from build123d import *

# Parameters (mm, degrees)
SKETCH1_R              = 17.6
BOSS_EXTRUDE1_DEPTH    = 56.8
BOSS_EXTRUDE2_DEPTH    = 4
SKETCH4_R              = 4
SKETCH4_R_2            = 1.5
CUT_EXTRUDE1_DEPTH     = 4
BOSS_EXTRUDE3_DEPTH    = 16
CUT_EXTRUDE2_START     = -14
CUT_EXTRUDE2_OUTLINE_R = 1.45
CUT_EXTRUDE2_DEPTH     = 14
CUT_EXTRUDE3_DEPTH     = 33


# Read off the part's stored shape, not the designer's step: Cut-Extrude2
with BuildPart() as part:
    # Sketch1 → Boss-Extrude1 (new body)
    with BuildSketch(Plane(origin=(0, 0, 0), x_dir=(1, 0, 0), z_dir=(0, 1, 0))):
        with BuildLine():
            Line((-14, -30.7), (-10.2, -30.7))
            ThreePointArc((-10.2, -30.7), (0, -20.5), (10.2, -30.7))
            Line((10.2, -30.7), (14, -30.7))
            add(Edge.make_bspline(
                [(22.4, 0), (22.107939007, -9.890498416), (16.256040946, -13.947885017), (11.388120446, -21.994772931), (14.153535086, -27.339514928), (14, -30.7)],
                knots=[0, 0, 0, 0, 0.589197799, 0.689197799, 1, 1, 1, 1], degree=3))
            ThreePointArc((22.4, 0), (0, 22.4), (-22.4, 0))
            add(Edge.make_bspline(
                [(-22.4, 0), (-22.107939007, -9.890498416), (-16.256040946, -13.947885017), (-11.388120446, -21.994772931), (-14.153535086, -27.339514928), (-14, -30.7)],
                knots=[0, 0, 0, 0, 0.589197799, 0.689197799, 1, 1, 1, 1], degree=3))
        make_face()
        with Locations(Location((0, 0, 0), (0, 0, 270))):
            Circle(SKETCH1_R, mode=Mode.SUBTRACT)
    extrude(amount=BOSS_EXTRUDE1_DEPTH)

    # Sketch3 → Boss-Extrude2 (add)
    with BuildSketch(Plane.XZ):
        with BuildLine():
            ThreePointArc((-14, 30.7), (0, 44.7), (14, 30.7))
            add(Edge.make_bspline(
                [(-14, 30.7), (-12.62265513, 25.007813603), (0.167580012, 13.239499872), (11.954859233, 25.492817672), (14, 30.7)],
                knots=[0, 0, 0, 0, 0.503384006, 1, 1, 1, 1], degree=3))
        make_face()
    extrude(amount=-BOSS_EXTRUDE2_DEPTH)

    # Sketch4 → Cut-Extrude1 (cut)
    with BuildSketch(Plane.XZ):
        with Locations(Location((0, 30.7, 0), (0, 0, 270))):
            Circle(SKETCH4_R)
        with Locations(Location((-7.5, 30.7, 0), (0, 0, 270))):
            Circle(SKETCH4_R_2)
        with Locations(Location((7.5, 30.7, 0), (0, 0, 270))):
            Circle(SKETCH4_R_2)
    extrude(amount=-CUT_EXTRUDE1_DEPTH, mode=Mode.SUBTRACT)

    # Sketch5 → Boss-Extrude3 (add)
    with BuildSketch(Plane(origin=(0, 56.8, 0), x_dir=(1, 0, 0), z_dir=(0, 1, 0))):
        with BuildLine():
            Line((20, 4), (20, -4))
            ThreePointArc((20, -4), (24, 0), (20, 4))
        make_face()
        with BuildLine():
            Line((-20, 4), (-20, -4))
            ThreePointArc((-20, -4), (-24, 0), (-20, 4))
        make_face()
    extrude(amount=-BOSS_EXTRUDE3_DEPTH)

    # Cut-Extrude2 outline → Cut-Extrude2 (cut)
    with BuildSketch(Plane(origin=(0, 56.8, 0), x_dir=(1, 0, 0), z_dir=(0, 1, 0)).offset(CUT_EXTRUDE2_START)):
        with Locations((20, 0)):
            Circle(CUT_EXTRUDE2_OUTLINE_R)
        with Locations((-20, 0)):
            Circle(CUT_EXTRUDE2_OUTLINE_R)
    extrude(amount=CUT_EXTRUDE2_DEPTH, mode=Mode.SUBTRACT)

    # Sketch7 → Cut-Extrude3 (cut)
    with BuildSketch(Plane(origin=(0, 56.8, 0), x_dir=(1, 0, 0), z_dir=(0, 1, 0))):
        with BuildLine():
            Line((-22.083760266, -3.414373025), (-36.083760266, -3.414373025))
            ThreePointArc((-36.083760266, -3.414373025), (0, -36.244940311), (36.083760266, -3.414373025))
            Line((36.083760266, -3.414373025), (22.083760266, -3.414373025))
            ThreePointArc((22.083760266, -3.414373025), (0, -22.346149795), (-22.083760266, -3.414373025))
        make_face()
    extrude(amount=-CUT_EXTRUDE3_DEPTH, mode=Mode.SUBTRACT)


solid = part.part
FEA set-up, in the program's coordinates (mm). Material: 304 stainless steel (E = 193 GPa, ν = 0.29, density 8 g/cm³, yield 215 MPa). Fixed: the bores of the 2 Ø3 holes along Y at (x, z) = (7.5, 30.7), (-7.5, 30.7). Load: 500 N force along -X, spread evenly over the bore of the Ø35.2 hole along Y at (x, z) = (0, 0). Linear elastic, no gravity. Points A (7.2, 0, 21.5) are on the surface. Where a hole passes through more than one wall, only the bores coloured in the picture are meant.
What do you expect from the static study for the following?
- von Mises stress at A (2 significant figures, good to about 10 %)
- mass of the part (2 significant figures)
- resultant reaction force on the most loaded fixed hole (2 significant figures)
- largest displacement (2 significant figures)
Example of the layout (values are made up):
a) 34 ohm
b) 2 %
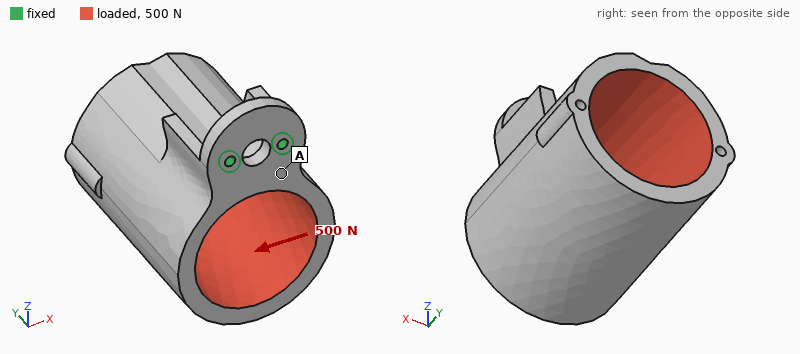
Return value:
a) 7.0 MPa
b) 300 g
c) 1.1 kN
d) 33 µm
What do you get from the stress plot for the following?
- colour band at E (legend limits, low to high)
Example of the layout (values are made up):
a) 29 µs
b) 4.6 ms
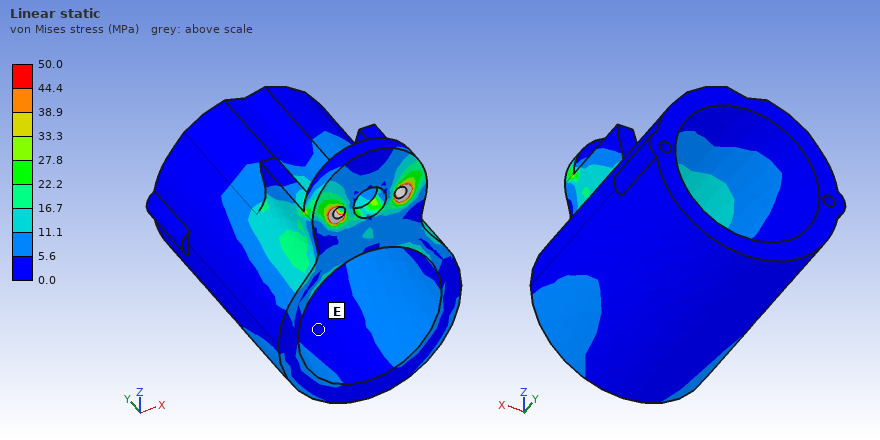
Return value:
a) 0.0 to 5.6 MPa
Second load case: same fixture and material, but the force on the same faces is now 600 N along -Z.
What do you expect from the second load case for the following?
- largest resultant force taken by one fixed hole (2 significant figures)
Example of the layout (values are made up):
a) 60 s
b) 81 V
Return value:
a) 300 N
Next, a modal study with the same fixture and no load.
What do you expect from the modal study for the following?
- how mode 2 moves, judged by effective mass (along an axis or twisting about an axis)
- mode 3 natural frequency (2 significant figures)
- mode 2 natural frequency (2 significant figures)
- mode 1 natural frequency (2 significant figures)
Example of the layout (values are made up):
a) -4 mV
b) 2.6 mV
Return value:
a) along X
b) 1800 Hz
c) 1400 Hz
d) 500 Hz
